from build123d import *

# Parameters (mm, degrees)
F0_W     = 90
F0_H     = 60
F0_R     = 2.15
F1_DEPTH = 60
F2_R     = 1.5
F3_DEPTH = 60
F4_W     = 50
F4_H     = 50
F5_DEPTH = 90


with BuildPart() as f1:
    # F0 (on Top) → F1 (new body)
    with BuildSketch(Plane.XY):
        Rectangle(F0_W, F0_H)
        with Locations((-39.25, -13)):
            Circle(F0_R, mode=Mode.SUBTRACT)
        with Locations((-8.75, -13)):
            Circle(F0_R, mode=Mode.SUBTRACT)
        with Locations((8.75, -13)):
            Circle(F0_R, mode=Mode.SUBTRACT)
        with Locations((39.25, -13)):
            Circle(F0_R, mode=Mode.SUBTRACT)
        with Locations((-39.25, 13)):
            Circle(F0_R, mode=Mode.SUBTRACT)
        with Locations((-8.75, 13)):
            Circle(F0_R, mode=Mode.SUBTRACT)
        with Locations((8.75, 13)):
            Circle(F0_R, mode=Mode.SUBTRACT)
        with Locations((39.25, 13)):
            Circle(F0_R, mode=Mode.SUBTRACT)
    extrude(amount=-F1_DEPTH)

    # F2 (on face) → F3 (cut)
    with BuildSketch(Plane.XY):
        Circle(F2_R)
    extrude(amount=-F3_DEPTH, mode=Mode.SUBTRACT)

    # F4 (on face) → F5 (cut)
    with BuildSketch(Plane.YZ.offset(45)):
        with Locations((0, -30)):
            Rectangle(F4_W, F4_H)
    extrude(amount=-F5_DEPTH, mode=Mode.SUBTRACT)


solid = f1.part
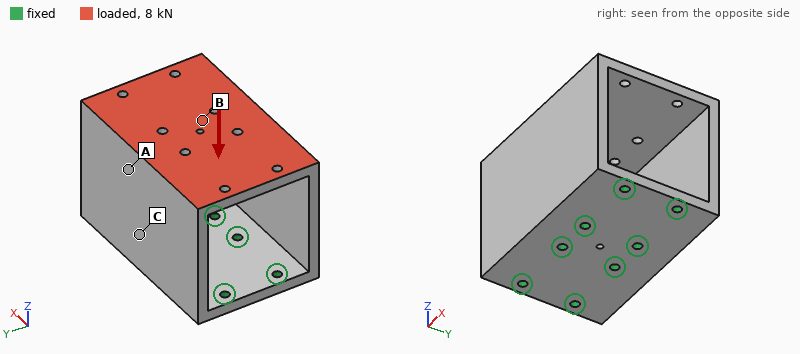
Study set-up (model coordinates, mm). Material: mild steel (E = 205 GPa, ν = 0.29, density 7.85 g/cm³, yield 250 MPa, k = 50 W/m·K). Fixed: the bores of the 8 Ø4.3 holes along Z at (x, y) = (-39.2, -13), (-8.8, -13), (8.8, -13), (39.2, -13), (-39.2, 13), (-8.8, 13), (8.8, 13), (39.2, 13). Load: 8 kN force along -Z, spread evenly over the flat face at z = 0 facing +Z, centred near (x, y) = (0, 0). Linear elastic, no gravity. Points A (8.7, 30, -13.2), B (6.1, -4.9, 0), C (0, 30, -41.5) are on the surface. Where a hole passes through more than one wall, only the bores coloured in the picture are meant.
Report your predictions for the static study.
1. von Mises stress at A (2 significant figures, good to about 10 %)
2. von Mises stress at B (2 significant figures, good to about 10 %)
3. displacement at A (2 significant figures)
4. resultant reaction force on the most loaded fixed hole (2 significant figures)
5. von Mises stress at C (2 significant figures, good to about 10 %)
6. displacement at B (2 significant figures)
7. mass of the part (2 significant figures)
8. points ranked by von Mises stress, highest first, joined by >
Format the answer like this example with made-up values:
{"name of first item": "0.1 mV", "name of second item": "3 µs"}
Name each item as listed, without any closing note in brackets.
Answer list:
{"von Mises stress at A": "32 MPa", "von Mises stress at B": "65 MPa", "displacement at A": "26 µm", "resultant reaction force on the most loaded fixed hole": "1.1 kN", "von Mises stress at C": "20 MPa", "displacement at B": "63 µm", "mass of the part": "770 g", "points ranked by von Mises stress, highest first, joined by >": "B > A > C"}
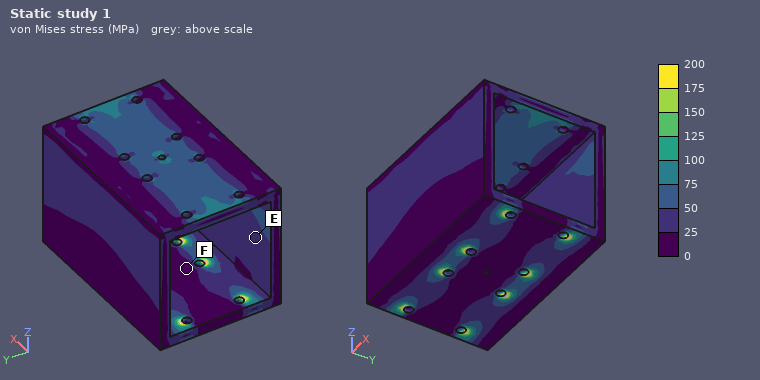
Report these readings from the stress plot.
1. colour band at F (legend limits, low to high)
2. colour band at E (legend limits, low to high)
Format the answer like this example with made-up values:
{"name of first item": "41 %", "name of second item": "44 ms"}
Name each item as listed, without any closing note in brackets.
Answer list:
{"colour band at F": "0 to 25 MPa", "colour band at E": "25 to 50 MPa"}
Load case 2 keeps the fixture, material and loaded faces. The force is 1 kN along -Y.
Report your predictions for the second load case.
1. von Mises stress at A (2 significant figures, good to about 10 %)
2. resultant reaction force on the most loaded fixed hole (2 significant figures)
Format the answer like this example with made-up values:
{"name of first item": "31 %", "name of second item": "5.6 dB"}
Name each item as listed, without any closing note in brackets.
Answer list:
{"von Mises stress at A": "20 MPa", "resultant reaction force on the most loaded fixed hole": "310 N"}
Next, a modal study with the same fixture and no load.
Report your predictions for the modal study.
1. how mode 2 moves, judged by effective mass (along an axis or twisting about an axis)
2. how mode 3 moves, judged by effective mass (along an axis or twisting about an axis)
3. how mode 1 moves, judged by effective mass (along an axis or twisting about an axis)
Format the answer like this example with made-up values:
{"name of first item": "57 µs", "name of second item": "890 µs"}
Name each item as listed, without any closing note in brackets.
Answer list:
{"how mode 2 moves, judged by effective mass": "along X", "how mode 3 moves, judged by effective mass": "twisting about Z", "how mode 1 moves, judged by effective mass": "along Y"}
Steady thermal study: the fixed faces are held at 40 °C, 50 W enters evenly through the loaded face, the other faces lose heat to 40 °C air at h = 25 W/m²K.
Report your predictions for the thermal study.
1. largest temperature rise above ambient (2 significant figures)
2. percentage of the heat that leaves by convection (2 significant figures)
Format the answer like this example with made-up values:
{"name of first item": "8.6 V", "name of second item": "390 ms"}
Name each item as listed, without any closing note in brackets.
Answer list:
{"largest temperature rise above ambient": "60 K", "percentage of the heat that leaves by convection": "46 %"}
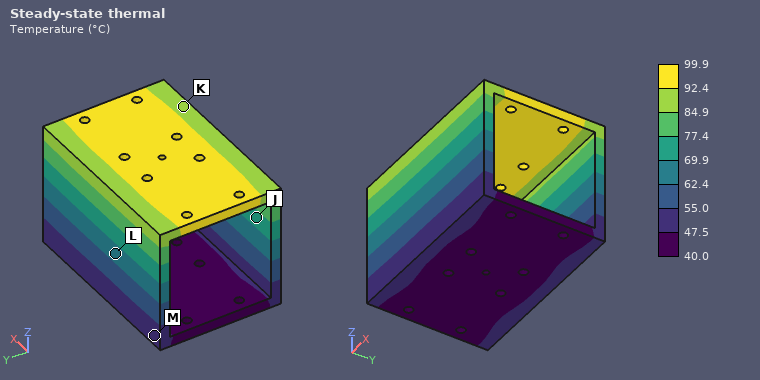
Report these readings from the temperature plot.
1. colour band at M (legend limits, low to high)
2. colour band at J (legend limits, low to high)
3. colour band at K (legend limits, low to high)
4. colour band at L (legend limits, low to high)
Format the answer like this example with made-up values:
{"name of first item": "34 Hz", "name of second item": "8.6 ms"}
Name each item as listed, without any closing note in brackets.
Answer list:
{"colour band at M": "47.5 to 55.0 °C", "colour band at J": "69.9 to 77.4 °C", "colour band at K": "84.9 to 92.4 °C", "colour band at L": "62.4 to 69.9 °C"}
